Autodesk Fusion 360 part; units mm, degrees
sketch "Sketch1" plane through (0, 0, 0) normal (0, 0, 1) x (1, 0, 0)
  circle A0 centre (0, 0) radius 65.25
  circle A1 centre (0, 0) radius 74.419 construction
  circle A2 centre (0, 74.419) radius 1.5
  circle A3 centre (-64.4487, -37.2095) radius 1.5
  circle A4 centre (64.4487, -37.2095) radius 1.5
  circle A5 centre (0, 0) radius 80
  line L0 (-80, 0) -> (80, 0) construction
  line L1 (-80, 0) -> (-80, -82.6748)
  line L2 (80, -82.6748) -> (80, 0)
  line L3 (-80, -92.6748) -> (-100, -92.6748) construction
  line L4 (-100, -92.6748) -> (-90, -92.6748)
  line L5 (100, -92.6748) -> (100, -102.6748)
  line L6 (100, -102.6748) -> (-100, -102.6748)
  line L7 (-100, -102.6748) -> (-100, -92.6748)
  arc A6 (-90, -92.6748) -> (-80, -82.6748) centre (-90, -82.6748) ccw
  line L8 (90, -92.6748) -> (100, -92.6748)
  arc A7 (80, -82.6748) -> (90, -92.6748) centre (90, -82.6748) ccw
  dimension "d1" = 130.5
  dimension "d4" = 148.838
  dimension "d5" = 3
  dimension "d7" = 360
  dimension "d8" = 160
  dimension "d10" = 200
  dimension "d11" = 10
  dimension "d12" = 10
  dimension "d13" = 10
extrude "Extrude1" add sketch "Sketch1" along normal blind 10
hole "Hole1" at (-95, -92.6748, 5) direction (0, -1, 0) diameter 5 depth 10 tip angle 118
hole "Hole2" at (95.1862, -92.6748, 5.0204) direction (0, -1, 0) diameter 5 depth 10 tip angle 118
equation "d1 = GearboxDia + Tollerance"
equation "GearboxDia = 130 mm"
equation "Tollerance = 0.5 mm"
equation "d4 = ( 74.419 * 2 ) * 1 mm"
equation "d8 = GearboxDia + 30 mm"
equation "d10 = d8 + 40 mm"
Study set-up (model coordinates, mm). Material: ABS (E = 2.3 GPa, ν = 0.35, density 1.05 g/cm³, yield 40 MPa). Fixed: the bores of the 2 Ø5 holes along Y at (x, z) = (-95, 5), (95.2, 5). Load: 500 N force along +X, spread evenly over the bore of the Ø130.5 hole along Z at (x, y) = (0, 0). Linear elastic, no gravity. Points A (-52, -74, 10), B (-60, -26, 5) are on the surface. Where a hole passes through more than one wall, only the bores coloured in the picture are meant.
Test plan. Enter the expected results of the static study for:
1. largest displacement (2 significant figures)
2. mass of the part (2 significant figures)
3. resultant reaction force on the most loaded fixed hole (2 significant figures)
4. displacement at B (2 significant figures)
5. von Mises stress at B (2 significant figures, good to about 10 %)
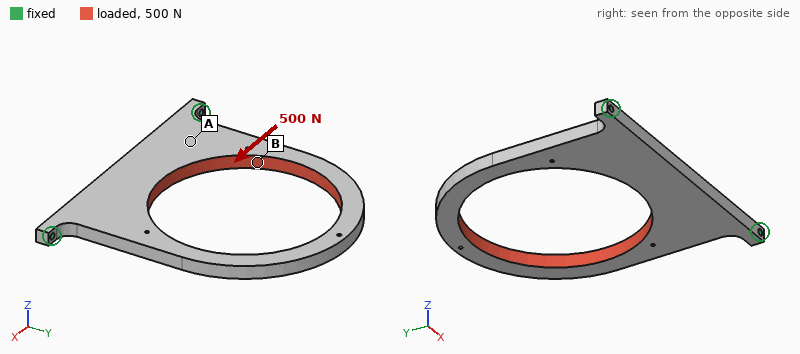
1.6 mm
140 g
370 N
0.28 mm
8.3 MPa
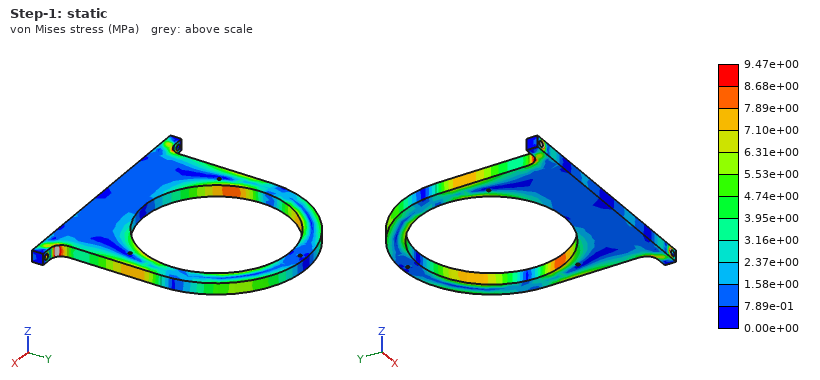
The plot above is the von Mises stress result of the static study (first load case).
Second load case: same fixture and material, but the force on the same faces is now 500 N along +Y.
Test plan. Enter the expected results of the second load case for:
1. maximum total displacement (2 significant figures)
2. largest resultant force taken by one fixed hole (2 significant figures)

0.30 mm
300 N
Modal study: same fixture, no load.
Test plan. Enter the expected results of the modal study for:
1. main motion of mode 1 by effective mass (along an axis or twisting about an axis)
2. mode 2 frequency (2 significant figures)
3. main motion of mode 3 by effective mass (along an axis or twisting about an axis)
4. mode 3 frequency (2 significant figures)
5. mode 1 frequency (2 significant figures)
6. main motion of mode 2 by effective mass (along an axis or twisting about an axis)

along Z
180 Hz
along Z
260 Hz
54 Hz
twisting about Y
